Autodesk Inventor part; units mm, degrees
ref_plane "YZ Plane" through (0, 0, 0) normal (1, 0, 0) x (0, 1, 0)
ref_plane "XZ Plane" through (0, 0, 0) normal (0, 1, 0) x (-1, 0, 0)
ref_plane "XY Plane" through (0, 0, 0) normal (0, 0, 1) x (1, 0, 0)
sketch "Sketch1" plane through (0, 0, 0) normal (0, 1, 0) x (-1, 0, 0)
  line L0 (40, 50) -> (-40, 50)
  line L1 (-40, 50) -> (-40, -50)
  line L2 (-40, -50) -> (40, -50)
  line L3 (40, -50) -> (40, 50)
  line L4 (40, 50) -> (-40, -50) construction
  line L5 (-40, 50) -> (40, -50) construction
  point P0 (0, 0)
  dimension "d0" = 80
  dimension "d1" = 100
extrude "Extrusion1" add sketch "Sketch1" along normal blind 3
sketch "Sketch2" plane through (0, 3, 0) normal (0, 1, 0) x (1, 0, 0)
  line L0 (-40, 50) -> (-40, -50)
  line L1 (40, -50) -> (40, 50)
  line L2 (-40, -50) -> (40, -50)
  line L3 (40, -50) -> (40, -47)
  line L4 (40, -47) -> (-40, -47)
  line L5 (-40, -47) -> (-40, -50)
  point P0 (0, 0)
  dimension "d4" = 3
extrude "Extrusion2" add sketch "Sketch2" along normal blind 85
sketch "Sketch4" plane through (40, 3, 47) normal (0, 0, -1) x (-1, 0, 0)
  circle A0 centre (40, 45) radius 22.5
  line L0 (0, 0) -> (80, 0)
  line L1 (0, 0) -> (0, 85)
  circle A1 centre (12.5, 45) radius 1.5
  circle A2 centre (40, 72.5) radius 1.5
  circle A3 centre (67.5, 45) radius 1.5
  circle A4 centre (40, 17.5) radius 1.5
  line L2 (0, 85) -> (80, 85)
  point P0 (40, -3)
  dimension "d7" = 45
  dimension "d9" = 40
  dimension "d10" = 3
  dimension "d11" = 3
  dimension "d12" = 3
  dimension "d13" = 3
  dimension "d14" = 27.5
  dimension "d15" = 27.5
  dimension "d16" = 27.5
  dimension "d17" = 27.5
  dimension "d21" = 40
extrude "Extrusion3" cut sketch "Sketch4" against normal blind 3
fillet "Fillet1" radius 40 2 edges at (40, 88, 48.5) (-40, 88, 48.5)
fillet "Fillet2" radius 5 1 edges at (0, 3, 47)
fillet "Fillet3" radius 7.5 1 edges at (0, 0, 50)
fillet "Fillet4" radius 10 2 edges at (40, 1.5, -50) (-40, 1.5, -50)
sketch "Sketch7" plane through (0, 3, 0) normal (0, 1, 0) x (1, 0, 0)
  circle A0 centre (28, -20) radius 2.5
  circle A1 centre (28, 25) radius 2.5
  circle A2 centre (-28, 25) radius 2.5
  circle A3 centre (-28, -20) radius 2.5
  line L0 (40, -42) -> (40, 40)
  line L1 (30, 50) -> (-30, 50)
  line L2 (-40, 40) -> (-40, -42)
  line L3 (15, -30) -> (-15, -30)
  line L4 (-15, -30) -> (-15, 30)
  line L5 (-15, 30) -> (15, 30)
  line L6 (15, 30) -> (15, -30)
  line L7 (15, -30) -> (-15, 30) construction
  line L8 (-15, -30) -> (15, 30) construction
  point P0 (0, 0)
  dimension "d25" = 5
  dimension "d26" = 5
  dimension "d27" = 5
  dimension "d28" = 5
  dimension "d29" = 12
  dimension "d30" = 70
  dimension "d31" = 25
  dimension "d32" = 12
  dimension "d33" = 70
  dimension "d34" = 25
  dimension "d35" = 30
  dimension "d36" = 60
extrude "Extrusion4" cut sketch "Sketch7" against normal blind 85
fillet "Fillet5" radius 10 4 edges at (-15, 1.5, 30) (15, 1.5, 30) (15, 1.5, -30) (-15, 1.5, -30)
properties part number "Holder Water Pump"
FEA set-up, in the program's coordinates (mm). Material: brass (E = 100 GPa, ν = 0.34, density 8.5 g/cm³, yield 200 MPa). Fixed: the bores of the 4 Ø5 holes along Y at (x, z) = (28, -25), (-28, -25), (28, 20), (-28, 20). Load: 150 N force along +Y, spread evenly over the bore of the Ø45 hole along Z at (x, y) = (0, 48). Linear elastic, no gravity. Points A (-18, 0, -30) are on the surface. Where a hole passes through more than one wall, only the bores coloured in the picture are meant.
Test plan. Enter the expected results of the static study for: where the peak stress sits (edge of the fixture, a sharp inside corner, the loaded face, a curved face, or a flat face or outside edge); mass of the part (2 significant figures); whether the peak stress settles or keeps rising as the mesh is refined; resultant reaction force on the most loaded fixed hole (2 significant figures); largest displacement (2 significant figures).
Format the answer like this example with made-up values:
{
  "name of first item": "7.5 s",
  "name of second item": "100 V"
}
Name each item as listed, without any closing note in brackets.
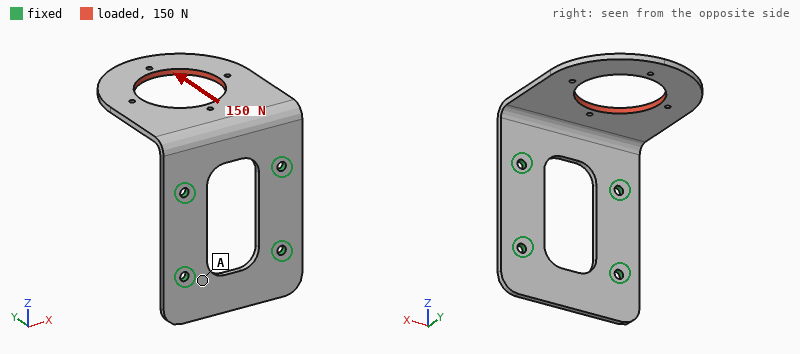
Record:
{
  "where the peak stress sits": "edge of the fixture",
  "mass of the part": "270 g",
  "whether the peak stress settles or keeps rising as the mesh is refined": "keeps rising",
  "resultant reaction force on the most loaded fixed hole": "79 N",
  "largest displacement": "0.38 mm"
}
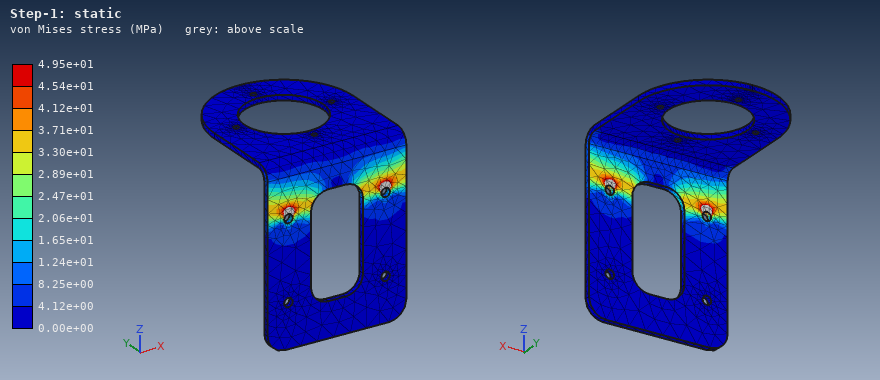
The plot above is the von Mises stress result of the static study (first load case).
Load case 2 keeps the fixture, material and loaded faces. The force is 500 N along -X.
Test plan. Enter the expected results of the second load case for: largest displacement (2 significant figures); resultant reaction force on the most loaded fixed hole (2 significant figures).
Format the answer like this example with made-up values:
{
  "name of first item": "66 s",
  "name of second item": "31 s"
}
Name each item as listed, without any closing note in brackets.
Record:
{
  "largest displacement": "0.61 mm",
  "resultant reaction force on the most loaded fixed hole": "500 N"
}
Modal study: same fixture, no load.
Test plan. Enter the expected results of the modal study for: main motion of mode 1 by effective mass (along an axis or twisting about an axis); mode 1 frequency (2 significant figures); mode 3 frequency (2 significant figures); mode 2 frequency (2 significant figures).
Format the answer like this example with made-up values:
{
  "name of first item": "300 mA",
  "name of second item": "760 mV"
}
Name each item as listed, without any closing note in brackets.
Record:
{
  "main motion of mode 1 by effective mass": "along Z",
  "mode 1 frequency": "180 Hz",
  "mode 3 frequency": "710 Hz",
  "mode 2 frequency": "460 Hz"
}
